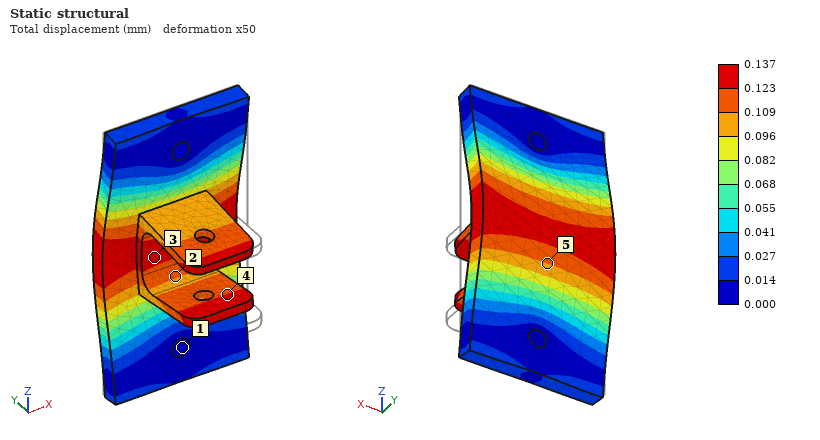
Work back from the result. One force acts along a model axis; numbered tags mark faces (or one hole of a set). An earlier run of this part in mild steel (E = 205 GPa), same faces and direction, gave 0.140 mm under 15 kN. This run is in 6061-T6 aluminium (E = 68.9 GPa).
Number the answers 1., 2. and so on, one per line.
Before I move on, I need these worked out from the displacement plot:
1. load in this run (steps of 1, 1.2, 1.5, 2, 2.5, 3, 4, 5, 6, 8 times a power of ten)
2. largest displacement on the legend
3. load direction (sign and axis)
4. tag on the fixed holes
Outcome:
1. 5 kN
2. 0.137 mm
3. +Y
4. 1
